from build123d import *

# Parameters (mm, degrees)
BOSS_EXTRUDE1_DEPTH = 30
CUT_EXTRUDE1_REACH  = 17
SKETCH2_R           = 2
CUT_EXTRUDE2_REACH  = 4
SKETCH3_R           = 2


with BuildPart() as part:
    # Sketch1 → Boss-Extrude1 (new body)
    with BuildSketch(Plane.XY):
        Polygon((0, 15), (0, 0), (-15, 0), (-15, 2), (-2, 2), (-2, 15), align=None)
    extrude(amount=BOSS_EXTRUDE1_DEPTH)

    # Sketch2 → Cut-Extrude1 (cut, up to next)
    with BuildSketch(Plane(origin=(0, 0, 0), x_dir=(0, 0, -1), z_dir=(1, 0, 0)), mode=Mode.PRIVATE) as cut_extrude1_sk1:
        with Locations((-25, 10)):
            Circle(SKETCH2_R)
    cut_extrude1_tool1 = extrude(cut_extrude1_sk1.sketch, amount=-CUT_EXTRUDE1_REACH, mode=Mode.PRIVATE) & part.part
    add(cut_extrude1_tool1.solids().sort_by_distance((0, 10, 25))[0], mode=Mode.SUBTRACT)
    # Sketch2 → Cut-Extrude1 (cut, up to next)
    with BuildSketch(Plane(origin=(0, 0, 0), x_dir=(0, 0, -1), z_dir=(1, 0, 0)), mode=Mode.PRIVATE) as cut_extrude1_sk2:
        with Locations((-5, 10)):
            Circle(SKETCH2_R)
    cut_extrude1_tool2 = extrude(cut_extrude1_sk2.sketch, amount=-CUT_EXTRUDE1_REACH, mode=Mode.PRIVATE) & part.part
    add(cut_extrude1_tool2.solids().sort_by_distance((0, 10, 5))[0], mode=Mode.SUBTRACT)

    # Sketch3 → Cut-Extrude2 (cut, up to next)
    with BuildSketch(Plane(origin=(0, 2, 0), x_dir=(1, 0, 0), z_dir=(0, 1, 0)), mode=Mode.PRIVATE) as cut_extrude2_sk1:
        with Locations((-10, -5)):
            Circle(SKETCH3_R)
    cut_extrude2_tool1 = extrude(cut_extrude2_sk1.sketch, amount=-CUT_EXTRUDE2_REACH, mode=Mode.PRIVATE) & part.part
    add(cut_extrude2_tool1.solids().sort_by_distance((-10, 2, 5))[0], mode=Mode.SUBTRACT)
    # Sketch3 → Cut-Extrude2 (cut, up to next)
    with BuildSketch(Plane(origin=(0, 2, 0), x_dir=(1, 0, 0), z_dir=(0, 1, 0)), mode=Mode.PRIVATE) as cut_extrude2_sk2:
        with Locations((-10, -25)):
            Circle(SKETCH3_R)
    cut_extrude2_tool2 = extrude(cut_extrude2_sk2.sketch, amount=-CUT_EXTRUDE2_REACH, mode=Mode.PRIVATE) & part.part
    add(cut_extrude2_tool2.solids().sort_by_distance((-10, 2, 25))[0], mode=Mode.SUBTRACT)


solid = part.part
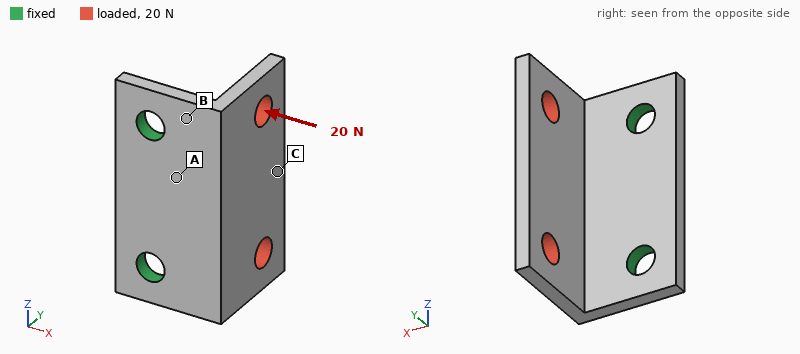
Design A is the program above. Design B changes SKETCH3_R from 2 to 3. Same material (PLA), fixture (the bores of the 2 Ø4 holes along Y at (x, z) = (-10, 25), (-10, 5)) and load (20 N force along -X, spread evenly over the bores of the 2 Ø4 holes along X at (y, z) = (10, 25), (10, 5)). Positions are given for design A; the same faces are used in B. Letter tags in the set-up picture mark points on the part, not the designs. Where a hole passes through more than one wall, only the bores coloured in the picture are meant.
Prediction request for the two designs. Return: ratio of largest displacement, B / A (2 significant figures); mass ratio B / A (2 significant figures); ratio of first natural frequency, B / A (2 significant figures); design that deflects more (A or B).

0.88
0.96
1.1
A
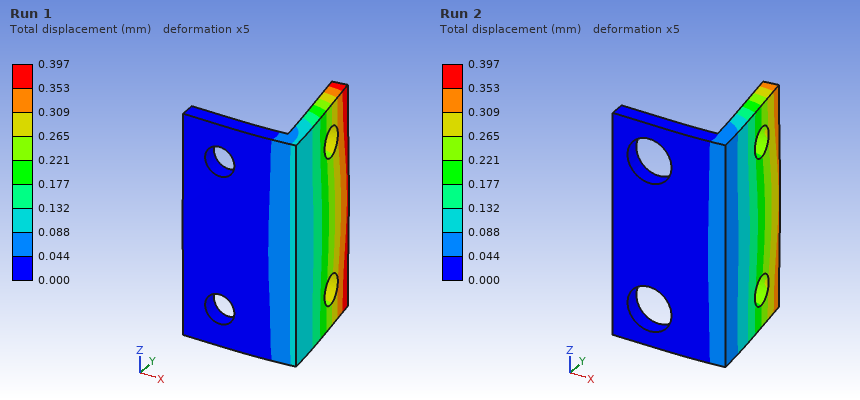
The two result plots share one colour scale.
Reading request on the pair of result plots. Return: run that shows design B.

Run 2
